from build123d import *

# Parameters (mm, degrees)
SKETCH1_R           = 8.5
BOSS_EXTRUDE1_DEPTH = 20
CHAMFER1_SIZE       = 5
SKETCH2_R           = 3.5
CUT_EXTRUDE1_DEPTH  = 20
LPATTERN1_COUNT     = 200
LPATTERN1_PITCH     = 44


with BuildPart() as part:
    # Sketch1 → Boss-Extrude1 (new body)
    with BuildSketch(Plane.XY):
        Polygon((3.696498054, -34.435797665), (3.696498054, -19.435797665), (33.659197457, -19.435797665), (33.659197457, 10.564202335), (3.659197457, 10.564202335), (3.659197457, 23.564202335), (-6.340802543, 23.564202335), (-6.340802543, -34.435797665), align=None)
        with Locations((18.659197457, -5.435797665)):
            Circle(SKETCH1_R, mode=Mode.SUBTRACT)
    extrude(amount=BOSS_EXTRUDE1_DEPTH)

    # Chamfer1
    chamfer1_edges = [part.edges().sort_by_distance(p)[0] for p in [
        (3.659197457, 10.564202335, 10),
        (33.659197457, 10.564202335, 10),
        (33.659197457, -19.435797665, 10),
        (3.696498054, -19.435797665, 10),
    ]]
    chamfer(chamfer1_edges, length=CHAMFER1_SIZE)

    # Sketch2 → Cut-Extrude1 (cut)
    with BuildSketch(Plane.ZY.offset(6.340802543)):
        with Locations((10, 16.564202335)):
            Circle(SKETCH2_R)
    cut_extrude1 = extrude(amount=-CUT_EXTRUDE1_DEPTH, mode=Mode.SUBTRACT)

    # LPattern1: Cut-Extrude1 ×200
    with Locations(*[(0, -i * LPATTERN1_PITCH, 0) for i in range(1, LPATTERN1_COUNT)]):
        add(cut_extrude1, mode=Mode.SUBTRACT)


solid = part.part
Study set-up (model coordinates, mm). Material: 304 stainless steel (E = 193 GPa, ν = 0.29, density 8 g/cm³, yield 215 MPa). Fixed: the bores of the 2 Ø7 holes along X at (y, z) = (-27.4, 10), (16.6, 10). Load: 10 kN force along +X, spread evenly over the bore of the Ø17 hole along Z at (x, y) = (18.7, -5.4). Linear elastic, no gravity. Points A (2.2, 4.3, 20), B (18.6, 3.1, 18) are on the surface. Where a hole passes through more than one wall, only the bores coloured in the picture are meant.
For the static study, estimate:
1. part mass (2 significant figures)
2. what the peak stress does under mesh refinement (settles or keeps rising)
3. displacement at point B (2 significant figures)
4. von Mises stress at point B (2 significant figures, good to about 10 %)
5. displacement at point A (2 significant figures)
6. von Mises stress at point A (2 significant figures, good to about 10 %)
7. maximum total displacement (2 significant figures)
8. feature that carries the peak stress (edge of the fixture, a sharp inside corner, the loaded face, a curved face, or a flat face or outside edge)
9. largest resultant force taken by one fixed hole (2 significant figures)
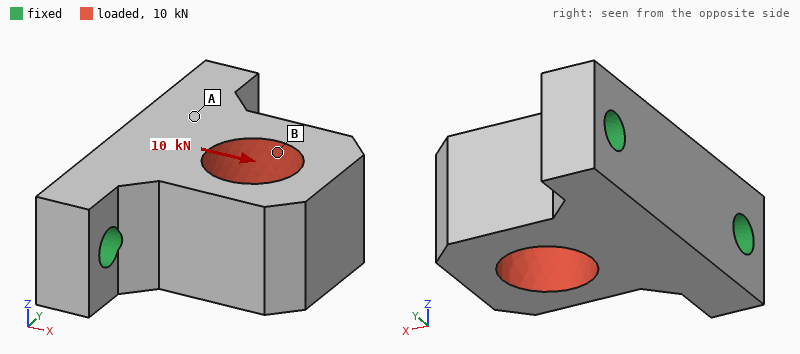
190 g
keeps rising
5.0 µm
35 MPa
3.8 µm
13 MPa
7.8 µm
edge of the fixture
5.4 kN
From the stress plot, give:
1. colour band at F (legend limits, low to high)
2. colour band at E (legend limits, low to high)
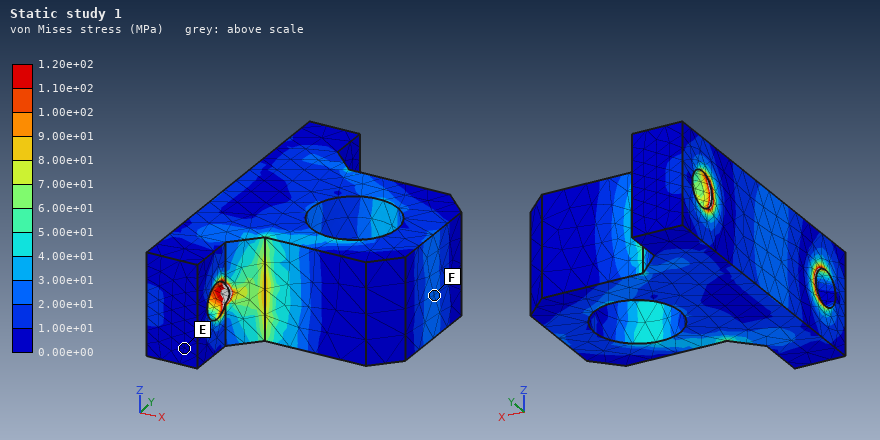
2.00e+01 to 3.00e+01 MPa
0.00e+00 to 1.00e+01 MPa
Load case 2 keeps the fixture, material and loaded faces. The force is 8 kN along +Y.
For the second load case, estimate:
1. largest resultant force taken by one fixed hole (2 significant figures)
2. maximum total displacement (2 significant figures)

5.7 kN
19 µm
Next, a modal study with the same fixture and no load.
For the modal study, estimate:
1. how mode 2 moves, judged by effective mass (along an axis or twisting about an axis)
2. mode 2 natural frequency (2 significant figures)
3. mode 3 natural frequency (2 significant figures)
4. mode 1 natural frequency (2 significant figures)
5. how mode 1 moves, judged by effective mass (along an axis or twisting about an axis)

along Y
12 kHz
17 kHz
6800 Hz
along Z
